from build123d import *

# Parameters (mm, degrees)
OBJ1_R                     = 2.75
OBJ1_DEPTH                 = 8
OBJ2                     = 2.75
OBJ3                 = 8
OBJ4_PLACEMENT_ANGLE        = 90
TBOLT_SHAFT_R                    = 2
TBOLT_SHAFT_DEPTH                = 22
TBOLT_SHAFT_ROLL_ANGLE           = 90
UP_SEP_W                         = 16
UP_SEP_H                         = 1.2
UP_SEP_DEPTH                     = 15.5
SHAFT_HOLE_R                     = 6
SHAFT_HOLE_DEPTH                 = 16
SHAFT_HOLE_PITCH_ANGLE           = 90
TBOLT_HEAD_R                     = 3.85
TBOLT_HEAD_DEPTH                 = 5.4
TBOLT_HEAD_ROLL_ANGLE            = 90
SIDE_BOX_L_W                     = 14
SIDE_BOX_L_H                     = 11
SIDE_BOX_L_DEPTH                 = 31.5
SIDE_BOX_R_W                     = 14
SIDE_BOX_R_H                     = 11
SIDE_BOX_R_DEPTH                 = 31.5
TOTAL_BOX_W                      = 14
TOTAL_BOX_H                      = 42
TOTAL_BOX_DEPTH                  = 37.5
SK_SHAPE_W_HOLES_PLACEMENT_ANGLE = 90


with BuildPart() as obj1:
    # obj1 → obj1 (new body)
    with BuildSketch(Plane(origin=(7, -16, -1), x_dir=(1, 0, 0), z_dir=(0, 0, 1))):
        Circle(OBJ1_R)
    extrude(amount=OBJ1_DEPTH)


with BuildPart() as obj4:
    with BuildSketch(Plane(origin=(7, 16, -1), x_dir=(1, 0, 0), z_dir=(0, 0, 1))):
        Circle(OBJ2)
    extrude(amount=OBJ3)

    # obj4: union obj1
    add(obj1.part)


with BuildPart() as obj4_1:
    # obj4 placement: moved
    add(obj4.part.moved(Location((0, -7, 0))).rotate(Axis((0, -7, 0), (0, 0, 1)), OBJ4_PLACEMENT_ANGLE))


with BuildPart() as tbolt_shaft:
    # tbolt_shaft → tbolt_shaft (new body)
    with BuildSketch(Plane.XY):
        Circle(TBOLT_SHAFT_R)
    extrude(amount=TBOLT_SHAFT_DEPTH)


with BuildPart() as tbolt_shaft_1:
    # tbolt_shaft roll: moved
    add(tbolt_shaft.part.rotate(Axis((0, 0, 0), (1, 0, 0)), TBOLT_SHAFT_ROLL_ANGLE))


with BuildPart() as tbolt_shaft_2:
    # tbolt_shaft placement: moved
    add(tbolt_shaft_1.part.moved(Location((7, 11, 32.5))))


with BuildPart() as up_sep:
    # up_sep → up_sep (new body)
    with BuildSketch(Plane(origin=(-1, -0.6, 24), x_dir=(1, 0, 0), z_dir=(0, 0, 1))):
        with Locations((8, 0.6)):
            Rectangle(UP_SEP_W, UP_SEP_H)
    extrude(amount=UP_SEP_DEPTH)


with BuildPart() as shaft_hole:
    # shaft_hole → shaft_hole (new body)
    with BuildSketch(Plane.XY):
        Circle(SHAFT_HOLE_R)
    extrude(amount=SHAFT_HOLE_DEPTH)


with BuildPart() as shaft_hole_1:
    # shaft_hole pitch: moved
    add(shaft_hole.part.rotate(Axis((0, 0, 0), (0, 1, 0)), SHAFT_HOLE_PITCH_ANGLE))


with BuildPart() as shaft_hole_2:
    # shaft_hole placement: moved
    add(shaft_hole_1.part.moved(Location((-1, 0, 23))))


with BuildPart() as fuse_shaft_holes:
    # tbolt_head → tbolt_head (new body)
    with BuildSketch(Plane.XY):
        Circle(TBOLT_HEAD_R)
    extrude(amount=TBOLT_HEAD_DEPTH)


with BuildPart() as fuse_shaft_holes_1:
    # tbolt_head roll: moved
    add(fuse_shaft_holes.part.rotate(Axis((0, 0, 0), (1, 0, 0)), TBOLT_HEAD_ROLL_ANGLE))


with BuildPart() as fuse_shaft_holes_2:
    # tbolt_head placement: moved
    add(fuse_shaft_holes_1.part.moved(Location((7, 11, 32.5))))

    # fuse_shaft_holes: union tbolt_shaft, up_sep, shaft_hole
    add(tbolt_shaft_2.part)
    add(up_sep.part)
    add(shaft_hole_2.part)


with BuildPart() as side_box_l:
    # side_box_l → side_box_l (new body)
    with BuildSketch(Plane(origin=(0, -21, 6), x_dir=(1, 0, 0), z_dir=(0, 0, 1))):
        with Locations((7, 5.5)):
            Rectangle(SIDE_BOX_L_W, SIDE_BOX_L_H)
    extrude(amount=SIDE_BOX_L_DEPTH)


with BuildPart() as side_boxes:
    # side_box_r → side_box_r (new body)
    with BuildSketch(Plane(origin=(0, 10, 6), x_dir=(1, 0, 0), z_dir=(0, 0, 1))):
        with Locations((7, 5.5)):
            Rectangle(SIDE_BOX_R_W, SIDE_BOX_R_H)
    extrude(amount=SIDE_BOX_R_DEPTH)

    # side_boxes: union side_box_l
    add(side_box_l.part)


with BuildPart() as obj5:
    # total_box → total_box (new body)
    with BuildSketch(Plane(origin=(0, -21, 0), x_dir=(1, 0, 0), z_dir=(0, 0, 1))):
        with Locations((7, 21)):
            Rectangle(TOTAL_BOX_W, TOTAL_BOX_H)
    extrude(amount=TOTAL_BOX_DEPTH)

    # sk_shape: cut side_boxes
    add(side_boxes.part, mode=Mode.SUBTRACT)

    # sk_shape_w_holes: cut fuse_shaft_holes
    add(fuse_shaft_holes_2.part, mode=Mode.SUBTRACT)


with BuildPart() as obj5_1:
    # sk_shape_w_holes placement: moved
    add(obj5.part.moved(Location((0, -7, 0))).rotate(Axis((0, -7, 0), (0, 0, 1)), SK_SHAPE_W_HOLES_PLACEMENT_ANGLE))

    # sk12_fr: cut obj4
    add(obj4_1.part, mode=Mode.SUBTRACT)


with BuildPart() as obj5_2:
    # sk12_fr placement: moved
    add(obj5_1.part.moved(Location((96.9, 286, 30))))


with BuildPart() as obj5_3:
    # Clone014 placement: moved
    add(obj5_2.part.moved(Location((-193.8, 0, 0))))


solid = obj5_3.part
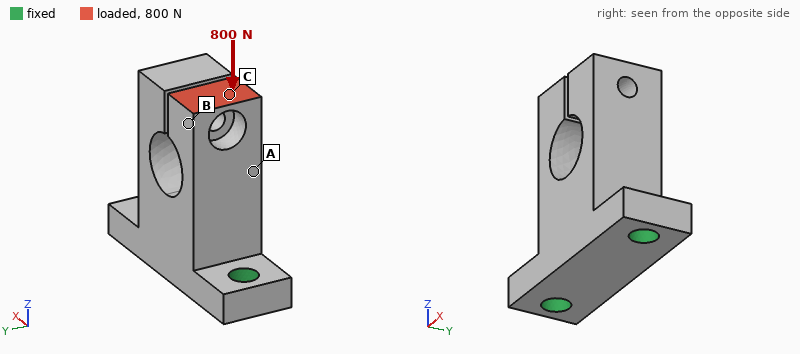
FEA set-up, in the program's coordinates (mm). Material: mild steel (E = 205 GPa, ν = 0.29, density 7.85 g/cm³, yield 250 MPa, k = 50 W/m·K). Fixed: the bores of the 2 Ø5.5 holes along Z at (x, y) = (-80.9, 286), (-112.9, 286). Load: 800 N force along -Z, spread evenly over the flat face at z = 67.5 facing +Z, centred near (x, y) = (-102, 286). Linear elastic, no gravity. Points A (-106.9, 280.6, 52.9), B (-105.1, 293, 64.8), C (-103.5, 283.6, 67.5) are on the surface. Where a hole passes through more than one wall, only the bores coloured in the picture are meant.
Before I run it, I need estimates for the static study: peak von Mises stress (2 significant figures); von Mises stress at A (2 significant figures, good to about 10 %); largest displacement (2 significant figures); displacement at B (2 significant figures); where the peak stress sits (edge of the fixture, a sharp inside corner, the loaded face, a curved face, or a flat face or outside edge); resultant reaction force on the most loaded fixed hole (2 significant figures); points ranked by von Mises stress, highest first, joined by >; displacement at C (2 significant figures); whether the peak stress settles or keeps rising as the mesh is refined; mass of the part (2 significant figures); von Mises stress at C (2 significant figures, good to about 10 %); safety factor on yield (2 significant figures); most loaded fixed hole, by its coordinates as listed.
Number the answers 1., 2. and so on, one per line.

1. 80 MPa
2. 37 MPa
3. 17 µm
4. 11 µm
5. a curved face
6. 590 N
7. A > C > B
8. 14 µm
9. settles
10. 78 g
11. 12 MPa
12. 3.1
13. (-112.9, 286)
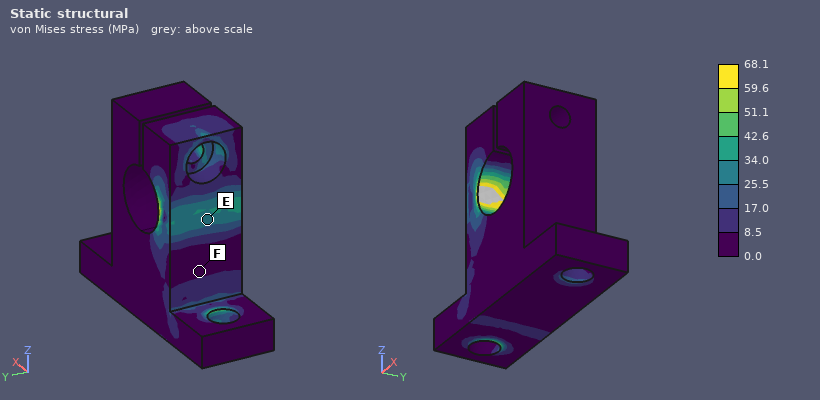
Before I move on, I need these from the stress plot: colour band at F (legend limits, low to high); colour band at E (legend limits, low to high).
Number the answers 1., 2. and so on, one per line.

1. 0.0 to 8.5 MPa
2. 25.5 to 34.0 MPa
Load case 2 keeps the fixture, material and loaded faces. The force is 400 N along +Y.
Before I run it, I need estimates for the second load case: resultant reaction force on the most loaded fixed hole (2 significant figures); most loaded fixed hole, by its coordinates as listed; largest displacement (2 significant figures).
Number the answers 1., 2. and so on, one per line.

1. 260 N
2. (-112.9, 286)
3. 41 µm
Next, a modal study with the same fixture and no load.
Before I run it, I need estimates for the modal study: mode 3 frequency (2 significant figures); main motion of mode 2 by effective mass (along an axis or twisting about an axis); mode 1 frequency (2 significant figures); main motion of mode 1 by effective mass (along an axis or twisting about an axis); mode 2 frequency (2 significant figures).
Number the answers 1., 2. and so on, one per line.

1. 6000 Hz
2. along X
3. 4400 Hz
4. along Y
5. 5500 Hz
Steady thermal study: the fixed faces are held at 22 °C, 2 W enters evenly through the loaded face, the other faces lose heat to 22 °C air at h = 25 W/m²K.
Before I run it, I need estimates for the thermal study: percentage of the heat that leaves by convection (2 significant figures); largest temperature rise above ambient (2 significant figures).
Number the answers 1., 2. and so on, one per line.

1. 20 %
2. 16 K
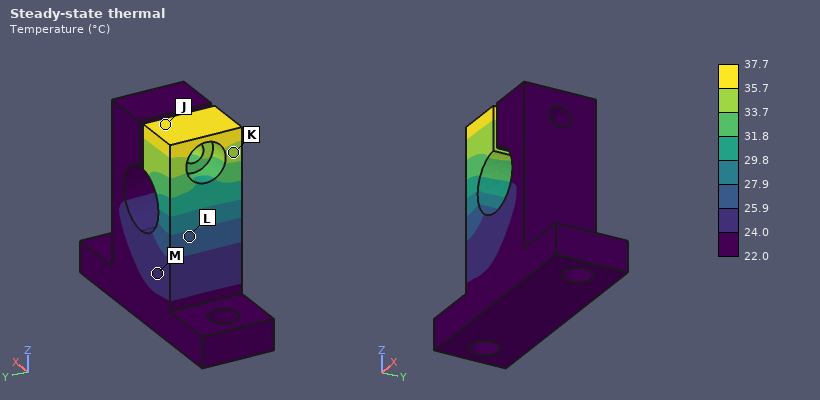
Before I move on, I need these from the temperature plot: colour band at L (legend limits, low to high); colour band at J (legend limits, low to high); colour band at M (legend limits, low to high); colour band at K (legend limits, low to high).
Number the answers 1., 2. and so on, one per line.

1. 25.9 to 27.9 °C
2. 35.7 to 37.7 °C
3. 24.0 to 25.9 °C
4. 33.7 to 35.7 °C
